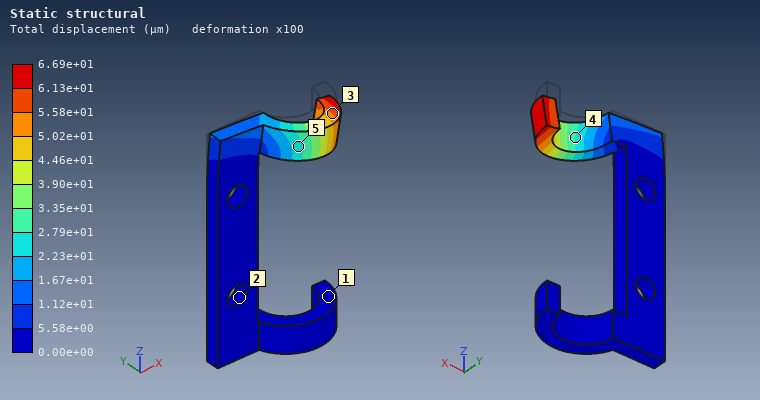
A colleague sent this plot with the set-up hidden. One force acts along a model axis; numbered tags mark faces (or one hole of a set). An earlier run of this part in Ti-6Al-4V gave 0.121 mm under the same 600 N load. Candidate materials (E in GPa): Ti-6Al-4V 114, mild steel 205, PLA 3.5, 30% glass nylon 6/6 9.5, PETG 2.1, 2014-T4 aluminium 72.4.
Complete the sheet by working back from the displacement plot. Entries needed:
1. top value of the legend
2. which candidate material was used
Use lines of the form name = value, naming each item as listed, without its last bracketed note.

top value of the legend = 6.69e+01 µm
which candidate material was used = mild steel
